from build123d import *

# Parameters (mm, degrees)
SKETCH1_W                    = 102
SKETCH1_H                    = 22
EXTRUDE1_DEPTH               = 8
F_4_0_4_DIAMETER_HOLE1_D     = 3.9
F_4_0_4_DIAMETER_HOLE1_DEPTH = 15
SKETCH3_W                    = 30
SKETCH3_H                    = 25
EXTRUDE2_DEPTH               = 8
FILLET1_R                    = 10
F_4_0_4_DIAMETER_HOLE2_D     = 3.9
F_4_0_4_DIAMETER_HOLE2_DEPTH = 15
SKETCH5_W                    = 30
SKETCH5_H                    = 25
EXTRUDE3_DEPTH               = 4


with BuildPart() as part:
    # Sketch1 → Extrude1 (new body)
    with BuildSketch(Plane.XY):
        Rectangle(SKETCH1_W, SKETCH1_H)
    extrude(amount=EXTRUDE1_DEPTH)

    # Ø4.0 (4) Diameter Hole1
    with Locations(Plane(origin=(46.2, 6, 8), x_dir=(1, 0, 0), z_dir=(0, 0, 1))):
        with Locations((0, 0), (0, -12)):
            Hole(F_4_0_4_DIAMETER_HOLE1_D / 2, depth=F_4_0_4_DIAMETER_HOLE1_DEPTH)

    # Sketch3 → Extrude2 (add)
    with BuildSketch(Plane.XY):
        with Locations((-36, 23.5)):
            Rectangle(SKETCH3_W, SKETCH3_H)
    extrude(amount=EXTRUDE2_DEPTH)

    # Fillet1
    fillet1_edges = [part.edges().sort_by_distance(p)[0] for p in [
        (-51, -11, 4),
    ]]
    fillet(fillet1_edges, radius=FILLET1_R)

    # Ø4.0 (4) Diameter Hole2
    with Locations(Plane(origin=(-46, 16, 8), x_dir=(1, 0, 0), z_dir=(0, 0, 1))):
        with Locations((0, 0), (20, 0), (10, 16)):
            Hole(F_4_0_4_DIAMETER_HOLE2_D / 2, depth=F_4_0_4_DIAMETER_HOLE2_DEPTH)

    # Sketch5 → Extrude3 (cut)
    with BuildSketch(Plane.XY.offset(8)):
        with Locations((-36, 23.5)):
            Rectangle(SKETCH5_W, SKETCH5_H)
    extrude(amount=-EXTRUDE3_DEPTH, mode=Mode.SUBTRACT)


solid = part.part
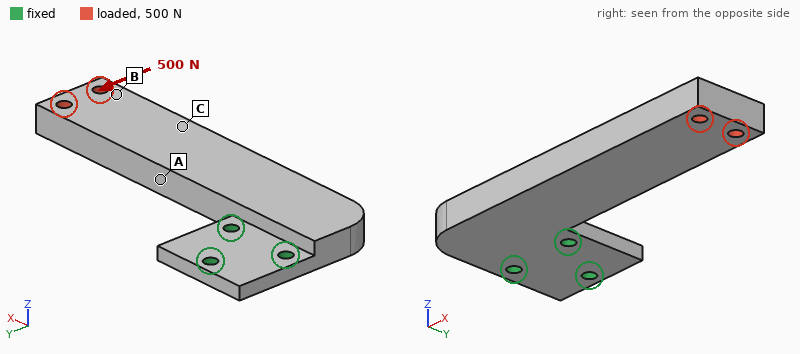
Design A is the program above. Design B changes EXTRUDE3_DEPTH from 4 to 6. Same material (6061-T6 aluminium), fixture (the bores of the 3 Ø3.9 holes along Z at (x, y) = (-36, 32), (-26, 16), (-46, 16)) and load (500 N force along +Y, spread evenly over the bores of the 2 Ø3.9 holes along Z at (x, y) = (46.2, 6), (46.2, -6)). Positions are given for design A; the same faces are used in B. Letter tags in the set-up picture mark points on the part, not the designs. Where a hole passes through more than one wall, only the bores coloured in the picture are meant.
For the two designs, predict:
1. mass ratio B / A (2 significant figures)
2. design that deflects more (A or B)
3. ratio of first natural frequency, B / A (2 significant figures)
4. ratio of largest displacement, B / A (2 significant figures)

0.93
B
0.74
1.7
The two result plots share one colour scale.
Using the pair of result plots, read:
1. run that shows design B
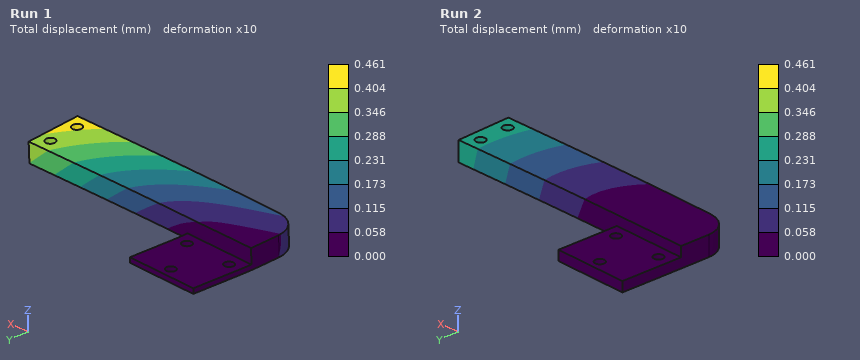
Run 1
